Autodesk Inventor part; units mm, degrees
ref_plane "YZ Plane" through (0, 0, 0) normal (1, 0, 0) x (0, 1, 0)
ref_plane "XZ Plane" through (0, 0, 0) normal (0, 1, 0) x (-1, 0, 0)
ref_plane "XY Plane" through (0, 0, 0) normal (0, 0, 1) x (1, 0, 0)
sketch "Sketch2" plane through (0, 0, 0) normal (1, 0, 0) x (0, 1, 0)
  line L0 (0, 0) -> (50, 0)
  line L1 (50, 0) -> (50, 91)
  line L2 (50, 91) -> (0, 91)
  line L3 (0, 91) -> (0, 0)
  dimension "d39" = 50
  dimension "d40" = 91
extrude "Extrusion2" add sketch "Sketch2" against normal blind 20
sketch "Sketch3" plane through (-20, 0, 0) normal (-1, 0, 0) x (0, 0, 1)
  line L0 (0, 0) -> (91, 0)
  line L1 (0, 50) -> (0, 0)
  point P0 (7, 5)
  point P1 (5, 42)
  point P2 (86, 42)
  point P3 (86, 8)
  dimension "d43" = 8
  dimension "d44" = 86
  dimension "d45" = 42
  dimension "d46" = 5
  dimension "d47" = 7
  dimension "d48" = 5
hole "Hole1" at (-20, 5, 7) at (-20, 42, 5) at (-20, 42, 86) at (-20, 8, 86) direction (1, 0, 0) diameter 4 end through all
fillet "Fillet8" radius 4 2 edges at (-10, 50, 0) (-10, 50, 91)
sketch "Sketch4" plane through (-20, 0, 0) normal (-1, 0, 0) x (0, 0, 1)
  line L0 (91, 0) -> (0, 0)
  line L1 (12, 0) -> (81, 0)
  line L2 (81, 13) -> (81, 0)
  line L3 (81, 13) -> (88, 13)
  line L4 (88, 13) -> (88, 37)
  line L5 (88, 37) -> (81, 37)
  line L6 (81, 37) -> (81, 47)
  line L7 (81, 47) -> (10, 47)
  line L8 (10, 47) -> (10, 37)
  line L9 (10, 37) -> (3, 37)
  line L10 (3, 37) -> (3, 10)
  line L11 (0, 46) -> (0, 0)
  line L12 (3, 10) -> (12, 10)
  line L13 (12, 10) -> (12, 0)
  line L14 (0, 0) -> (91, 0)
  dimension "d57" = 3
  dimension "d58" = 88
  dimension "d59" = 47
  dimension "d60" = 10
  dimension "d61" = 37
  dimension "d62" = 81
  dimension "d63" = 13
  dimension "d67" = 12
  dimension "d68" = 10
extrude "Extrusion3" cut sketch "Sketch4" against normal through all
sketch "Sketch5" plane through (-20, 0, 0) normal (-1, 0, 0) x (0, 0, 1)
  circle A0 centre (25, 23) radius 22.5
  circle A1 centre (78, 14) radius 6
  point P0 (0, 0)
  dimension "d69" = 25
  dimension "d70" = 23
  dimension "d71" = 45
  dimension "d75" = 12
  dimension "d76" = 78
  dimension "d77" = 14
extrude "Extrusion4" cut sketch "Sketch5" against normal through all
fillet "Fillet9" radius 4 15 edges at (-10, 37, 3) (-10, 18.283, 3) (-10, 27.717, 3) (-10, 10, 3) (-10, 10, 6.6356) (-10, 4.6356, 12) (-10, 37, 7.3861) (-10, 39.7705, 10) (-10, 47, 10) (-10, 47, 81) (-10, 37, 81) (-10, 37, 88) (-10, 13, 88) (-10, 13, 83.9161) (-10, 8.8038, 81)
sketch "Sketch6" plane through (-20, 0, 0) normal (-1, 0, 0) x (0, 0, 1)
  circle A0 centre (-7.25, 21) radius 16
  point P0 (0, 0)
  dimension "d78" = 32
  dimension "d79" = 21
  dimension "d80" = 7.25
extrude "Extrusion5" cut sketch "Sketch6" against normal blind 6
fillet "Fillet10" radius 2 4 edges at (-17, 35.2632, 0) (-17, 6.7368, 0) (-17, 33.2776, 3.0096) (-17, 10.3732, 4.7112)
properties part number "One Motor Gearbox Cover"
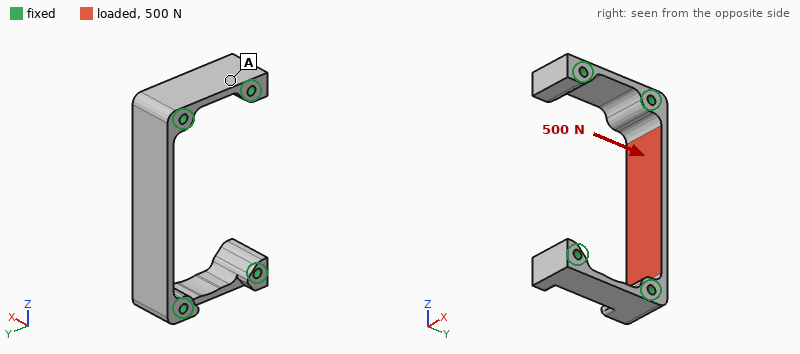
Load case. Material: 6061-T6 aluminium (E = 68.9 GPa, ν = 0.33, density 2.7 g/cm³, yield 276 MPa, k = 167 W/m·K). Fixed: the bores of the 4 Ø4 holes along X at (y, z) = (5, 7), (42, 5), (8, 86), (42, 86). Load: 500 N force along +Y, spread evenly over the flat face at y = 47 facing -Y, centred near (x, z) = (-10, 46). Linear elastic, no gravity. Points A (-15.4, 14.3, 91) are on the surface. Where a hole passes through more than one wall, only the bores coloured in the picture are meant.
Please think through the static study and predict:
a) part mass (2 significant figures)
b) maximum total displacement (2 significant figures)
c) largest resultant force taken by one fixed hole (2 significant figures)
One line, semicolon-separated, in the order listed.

42 g; 0.16 mm; 370 N
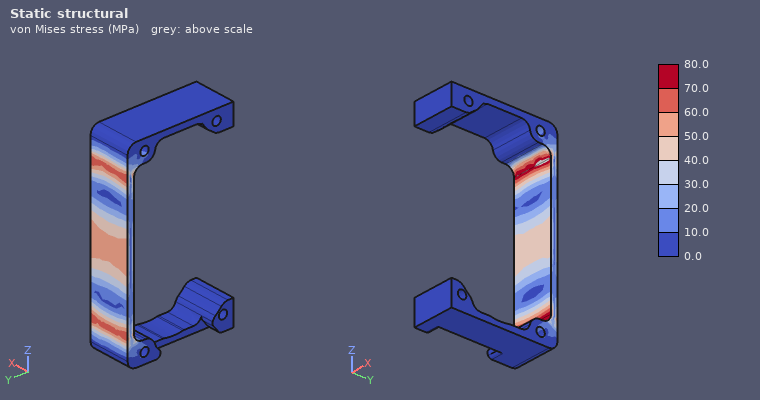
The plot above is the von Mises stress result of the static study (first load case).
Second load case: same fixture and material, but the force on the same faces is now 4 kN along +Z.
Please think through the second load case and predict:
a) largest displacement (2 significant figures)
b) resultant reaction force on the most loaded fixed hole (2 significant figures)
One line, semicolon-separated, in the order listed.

20 µm; 2.0 kN
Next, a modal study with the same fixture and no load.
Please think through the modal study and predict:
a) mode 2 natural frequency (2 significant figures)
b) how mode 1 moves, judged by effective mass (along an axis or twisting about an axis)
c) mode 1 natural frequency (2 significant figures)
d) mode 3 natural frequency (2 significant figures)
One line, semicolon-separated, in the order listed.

7300 Hz; along Y; 3200 Hz; 8500 Hz
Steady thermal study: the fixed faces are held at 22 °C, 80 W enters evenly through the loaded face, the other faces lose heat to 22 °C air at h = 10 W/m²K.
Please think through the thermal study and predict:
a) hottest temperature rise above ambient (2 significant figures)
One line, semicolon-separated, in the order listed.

87 K
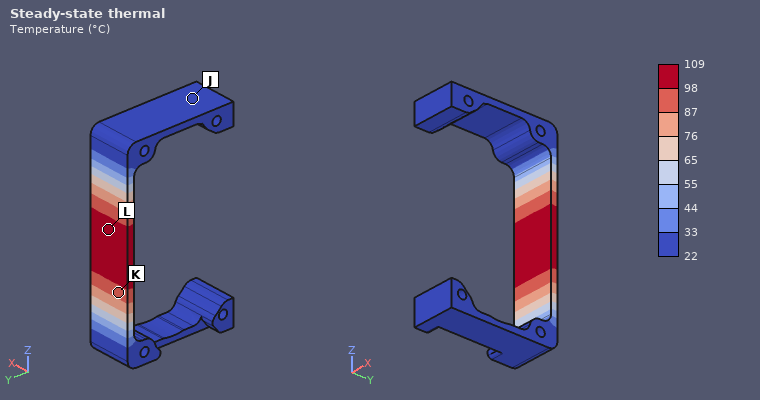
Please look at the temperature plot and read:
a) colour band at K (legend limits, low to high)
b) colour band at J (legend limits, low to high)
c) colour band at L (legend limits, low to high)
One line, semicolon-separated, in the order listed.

87 to 98 °C; 22 to 33 °C; 98 to 109 °C
